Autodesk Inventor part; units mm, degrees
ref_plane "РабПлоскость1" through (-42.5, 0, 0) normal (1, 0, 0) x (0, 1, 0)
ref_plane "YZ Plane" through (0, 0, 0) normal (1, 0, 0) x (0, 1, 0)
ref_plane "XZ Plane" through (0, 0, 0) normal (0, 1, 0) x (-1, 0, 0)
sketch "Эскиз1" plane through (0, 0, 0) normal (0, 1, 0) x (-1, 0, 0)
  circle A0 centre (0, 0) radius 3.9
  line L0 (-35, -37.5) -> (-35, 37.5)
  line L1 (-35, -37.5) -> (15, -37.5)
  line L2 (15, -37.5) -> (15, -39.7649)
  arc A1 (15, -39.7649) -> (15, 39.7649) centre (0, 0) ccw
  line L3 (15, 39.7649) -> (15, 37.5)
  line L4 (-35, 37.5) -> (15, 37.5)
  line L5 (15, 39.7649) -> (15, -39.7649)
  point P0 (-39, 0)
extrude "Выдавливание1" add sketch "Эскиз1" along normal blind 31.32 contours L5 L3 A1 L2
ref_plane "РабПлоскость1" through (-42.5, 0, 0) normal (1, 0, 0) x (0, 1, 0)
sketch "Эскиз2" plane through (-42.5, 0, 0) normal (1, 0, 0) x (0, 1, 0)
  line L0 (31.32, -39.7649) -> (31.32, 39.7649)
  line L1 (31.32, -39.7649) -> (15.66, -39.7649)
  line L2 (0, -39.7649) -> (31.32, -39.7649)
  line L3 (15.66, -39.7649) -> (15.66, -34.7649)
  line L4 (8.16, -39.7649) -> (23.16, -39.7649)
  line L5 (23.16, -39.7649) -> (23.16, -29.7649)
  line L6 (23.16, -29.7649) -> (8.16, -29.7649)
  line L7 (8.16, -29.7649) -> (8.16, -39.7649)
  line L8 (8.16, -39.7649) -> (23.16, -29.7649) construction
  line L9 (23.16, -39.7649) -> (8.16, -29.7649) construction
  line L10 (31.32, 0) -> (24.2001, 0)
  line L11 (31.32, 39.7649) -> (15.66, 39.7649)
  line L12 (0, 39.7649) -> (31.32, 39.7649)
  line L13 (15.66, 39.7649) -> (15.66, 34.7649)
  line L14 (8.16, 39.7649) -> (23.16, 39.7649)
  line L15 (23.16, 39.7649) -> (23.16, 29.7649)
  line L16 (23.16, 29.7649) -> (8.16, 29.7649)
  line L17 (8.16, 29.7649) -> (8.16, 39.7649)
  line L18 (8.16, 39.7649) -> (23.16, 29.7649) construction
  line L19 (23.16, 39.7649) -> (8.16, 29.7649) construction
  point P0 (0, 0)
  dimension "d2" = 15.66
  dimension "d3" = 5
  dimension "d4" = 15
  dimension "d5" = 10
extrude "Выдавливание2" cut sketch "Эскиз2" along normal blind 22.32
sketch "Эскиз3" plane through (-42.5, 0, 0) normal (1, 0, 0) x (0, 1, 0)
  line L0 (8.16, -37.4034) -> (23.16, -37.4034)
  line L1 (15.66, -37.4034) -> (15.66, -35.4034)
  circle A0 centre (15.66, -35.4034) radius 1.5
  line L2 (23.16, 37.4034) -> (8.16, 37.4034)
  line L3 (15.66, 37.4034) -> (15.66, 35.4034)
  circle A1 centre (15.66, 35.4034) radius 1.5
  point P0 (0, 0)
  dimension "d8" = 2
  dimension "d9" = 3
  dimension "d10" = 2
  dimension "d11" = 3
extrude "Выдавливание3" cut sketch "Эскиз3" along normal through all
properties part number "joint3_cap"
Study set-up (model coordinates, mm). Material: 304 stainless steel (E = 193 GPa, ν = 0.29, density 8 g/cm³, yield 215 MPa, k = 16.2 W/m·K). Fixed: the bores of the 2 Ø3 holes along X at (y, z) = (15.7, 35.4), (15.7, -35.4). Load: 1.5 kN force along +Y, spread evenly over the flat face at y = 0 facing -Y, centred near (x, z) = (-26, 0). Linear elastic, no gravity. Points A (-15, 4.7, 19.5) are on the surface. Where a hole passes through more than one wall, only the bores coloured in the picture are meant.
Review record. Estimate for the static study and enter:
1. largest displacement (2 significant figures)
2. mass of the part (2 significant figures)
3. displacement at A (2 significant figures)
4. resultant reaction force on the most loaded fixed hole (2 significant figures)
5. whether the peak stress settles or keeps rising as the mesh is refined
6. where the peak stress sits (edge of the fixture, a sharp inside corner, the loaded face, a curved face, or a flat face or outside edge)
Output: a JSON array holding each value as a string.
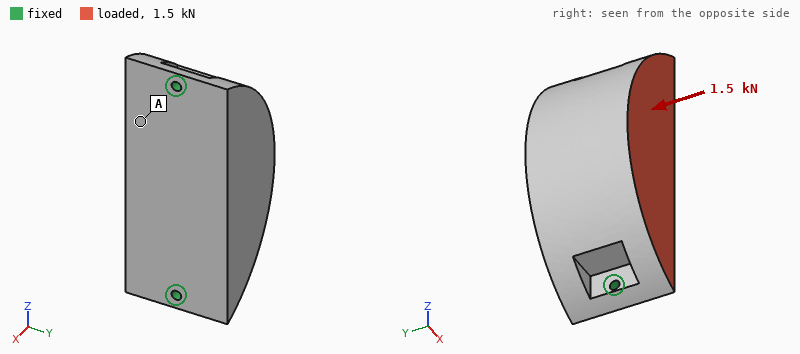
["24 µm", "390 g", "8.1 µm", "750 N", "keeps rising", "edge of the fixture"]
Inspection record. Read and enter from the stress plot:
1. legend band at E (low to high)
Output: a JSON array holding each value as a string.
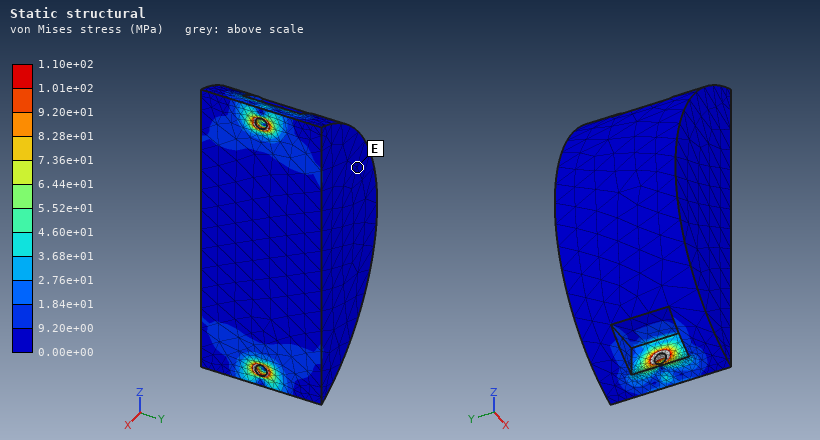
["0.00e+00 to 9.20e+00 MPa"]
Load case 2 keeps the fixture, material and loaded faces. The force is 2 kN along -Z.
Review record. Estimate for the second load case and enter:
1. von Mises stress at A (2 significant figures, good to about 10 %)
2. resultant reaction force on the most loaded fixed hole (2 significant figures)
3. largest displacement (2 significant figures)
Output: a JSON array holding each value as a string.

["5.7 MPa", "1.1 kN", "1.8 µm"]
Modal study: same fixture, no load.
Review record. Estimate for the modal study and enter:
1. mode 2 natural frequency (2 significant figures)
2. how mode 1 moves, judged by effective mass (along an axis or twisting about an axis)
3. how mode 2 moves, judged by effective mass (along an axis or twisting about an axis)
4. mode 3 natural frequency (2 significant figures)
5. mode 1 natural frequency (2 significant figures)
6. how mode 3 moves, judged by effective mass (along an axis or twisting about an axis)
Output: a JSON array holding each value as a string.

["6600 Hz", "along Y", "along X", "10 kHz", "2300 Hz", "along Z"]
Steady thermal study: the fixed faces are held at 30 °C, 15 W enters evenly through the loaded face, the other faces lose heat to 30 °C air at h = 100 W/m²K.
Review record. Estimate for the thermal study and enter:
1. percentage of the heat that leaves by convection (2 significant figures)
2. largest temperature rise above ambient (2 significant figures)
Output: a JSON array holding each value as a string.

["69 %", "24 K"]
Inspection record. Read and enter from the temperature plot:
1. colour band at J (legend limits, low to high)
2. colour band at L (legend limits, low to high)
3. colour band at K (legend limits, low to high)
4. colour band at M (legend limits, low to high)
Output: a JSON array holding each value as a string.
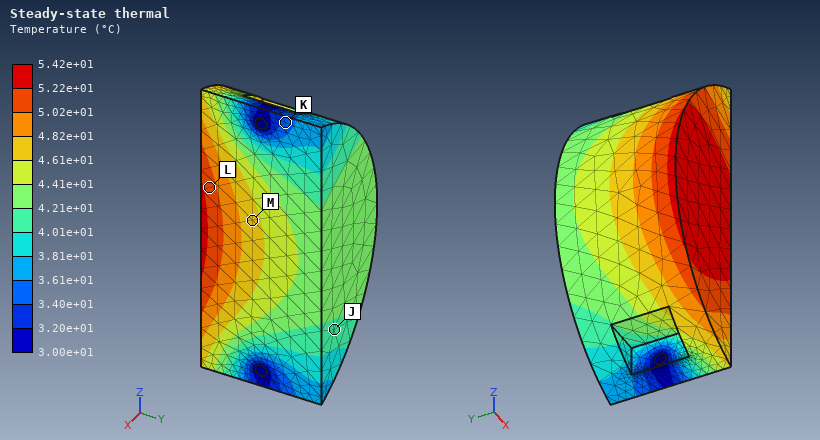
["4.01e+01 to 4.21e+01 °C", "5.02e+01 to 5.22e+01 °C", "3.40e+01 to 3.61e+01 °C", "4.61e+01 to 4.82e+01 °C"]
